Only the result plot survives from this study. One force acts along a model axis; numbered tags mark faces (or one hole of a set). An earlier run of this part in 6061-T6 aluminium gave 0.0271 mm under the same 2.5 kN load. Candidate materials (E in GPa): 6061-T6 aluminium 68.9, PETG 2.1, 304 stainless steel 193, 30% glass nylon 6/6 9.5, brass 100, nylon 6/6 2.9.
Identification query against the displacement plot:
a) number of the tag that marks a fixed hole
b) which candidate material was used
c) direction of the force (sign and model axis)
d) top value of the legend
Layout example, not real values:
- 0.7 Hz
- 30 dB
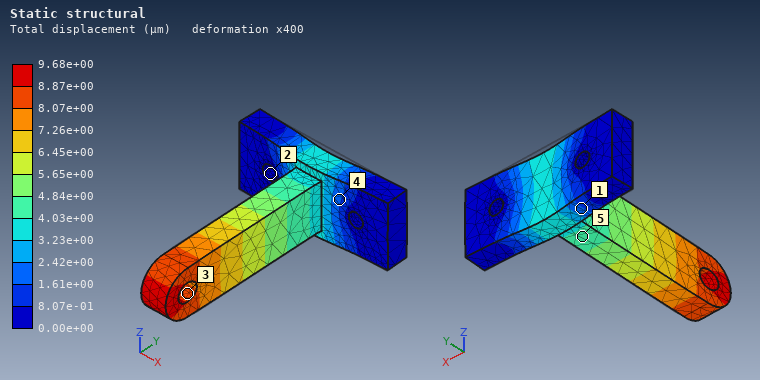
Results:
- 2
- 304 stainless steel
- -Y
- 9.68e+00 µm
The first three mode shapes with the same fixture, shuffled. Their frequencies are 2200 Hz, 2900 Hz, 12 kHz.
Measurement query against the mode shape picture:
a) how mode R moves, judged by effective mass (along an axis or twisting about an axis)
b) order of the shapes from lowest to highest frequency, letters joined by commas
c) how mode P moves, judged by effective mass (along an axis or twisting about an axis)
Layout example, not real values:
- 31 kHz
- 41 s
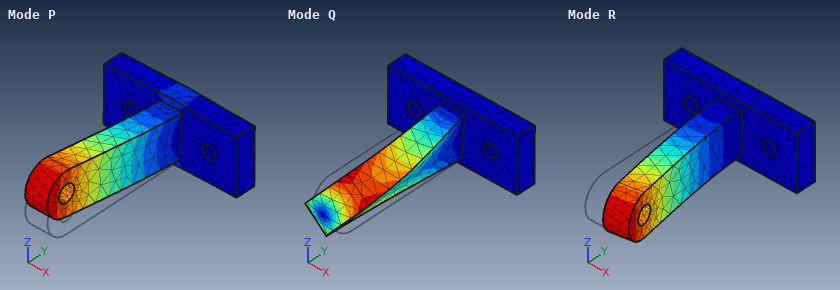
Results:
- along X
- R, P, Q
- along Z
